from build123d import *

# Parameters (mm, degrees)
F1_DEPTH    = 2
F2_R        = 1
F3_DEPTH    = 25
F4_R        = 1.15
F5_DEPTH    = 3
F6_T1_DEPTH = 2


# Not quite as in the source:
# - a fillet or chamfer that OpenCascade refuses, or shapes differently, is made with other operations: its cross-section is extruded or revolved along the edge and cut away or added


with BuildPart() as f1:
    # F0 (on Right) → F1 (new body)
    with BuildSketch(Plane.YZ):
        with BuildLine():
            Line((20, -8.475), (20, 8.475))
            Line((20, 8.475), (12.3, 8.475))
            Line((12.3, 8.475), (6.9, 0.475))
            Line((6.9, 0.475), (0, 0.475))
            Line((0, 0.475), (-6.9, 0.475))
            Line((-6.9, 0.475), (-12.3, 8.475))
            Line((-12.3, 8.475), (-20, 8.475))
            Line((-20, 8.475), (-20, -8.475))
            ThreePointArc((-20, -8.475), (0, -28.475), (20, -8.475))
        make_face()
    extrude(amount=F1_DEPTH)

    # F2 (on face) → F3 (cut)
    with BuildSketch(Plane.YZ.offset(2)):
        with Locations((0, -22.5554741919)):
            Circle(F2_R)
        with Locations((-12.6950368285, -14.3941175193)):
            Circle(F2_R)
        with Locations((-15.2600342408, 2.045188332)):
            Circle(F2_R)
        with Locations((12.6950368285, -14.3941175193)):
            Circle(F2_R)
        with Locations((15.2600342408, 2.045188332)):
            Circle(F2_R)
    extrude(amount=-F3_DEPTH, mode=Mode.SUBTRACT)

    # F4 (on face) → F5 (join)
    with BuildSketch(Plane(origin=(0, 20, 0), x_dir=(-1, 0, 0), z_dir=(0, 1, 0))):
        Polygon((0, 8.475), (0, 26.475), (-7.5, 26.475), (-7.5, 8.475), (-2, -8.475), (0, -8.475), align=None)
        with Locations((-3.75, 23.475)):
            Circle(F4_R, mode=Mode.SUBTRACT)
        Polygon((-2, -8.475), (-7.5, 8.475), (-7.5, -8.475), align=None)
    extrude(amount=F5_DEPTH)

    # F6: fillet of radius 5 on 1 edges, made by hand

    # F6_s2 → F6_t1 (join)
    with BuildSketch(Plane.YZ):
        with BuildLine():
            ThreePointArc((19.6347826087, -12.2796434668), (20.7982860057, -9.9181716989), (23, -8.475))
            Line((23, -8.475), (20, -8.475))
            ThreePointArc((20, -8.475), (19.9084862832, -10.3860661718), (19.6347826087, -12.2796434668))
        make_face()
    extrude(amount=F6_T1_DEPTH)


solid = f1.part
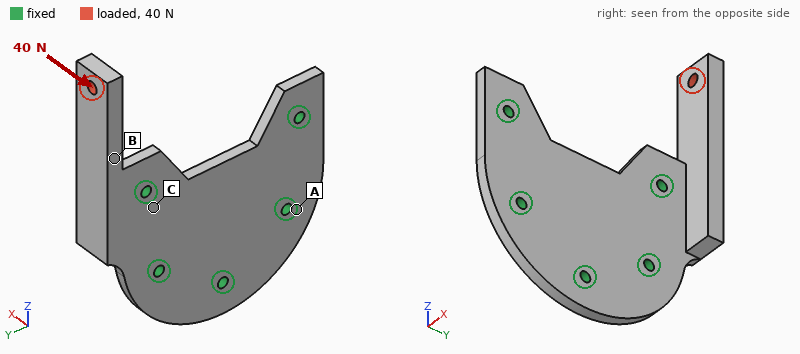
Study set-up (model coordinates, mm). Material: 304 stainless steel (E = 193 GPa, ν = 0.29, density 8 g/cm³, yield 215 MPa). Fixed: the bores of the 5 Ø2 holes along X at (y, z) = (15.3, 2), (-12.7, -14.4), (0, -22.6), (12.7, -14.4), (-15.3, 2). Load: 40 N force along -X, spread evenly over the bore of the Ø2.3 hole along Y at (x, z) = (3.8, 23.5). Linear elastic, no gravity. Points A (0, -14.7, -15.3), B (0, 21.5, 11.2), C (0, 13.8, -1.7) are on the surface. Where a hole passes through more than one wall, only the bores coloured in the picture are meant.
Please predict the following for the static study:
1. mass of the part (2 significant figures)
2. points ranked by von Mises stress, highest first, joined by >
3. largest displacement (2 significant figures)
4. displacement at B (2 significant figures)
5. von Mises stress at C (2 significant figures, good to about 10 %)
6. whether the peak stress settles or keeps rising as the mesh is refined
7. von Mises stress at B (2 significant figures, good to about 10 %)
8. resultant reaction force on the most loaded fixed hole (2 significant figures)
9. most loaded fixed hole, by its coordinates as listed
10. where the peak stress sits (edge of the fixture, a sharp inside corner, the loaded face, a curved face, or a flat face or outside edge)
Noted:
24 g
B > C > A
29 µm
11 µm
9.8 MPa
keeps rising
17 MPa
83 N
(15.3, 2)
edge of the fixture
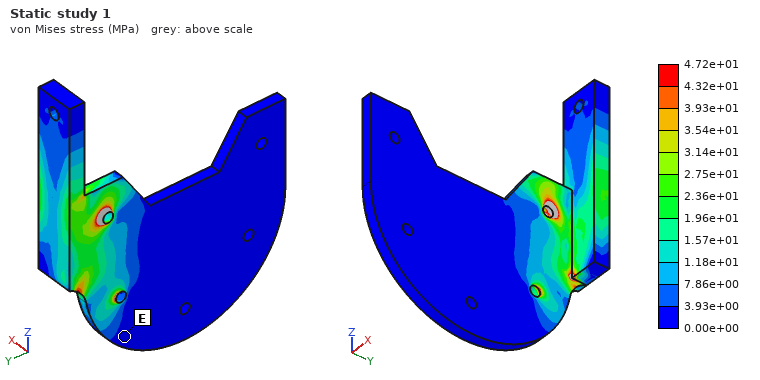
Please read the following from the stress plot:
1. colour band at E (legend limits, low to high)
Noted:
0.00e+00 to 3.93e+00 MPa
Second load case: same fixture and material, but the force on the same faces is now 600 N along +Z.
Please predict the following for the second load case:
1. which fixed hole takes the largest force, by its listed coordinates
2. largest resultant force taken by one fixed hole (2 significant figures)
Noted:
(15.3, 2)
480 N
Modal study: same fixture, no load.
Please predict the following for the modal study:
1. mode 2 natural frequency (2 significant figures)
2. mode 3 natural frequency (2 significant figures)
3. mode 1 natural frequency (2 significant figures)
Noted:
5400 Hz
9300 Hz
4300 Hz
